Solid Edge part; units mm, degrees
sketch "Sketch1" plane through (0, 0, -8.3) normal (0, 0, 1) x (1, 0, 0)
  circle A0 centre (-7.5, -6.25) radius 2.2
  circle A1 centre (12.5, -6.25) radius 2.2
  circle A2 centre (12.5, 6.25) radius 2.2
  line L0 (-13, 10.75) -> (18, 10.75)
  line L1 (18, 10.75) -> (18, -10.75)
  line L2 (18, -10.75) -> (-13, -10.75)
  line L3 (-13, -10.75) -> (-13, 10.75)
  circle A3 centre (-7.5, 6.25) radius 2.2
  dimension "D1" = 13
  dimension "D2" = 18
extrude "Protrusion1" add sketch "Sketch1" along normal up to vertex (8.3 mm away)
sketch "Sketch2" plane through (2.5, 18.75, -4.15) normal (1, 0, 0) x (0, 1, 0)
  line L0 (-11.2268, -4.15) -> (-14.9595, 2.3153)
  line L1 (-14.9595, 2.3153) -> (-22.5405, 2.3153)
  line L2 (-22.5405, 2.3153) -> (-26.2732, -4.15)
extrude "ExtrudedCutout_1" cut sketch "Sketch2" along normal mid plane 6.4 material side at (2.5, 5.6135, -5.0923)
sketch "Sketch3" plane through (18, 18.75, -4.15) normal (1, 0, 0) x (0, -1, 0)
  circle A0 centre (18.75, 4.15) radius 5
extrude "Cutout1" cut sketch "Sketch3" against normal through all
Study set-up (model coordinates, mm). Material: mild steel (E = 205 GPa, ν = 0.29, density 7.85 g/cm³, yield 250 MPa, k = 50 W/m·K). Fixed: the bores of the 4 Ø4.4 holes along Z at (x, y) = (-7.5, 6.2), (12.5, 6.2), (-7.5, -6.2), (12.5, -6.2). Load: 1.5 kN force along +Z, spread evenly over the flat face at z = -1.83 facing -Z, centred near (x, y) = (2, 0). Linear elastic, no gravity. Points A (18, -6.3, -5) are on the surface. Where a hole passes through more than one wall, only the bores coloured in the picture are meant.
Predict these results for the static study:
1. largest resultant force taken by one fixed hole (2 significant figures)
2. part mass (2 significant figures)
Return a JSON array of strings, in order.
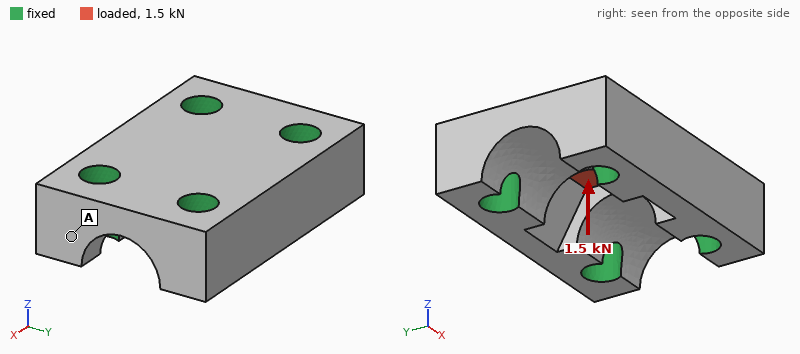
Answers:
["440 N", "28 g"]
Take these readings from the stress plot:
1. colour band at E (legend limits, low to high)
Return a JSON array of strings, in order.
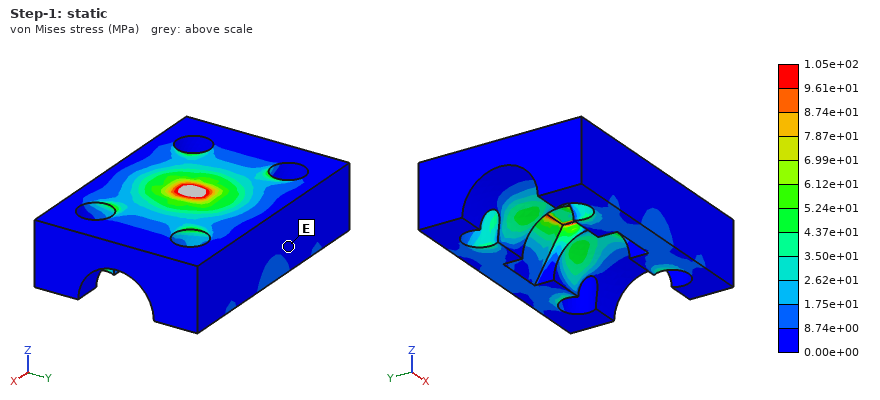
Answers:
["0.00e+00 to 8.74e+00 MPa"]
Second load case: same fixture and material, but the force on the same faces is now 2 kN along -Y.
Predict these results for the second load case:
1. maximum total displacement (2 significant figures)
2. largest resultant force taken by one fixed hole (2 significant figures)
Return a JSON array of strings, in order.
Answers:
["2.7 µm", "540 N"]
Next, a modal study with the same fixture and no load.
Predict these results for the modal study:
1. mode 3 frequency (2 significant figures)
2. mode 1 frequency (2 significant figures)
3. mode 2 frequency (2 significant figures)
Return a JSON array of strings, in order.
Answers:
["80 kHz", "74 kHz", "75 kHz"]
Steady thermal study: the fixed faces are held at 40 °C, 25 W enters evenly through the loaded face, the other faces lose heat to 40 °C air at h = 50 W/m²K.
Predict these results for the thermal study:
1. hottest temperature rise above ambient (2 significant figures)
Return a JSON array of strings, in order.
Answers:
["52 K"]
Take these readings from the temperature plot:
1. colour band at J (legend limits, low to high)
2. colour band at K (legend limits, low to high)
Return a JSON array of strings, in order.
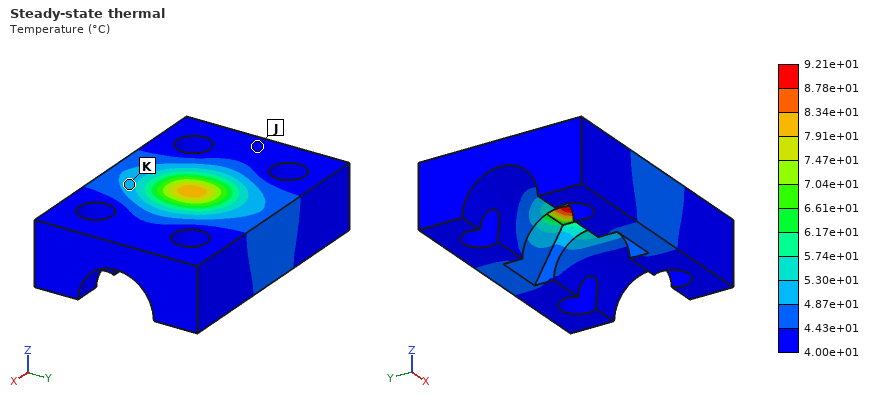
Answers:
["4.00e+01 to 4.43e+01 °C", "4.87e+01 to 5.30e+01 °C"]
